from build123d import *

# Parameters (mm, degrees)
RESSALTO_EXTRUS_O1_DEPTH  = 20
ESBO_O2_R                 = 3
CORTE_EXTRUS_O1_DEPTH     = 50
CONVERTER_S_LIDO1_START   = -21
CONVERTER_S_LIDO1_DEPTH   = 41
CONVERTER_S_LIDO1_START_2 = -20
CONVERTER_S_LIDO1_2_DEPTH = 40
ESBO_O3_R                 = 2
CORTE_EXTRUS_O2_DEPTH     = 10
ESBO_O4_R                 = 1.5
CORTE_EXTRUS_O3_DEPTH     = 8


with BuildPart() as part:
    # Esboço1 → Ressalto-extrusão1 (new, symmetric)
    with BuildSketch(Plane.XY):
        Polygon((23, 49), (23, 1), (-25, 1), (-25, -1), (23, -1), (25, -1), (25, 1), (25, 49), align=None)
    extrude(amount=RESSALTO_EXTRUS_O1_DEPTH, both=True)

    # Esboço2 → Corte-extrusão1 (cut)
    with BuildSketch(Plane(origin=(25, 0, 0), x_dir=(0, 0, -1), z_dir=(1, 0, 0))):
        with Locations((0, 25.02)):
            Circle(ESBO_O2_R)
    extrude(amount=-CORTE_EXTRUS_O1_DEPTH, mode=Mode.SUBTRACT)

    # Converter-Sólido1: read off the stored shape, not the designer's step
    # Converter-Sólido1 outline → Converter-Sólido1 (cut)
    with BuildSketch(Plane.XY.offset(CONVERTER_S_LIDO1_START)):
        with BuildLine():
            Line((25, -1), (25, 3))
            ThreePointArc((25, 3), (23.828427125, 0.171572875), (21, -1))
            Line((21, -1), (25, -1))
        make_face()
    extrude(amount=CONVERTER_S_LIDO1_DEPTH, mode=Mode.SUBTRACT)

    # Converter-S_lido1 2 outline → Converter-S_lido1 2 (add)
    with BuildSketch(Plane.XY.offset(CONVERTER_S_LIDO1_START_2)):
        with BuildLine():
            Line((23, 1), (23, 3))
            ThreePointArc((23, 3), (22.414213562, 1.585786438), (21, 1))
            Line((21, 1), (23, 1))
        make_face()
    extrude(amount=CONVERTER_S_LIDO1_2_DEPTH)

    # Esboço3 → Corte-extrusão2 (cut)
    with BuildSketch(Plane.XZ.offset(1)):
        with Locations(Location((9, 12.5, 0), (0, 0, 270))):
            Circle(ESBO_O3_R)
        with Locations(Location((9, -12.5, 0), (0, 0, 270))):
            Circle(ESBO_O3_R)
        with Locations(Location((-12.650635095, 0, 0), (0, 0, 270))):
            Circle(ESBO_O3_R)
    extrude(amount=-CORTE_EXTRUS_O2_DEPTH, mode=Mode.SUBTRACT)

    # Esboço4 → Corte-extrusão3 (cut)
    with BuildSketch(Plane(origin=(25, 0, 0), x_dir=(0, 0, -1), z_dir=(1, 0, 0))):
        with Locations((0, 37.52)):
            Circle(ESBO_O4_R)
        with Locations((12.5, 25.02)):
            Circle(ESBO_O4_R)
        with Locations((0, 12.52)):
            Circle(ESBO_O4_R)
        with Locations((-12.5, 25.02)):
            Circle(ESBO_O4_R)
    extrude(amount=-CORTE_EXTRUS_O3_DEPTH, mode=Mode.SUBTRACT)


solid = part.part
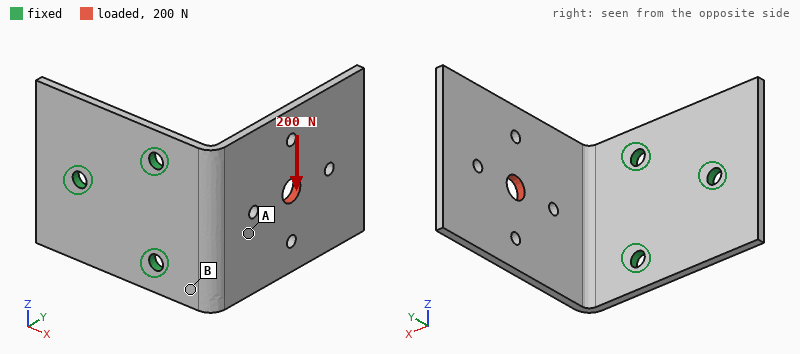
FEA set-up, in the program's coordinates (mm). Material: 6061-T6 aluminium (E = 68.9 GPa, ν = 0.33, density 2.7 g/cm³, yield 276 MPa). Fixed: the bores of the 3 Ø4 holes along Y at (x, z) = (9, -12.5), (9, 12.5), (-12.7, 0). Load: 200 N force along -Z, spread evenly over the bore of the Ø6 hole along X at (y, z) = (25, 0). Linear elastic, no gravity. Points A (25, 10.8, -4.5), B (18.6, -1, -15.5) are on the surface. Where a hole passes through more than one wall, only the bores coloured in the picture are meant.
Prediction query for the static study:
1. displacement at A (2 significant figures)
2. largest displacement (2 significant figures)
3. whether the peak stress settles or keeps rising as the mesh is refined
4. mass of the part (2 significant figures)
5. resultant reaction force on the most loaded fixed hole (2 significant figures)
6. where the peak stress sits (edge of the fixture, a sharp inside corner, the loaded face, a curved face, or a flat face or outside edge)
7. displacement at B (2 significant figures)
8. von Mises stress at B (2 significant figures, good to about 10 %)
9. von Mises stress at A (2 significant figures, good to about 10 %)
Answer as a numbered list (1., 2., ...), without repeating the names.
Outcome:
1. 0.086 mm
2. 0.42 mm
3. keeps rising
4. 20 g
5. 230 N
6. edge of the fixture
7. 0.064 mm
8. 43 MPa
9. 14 MPa
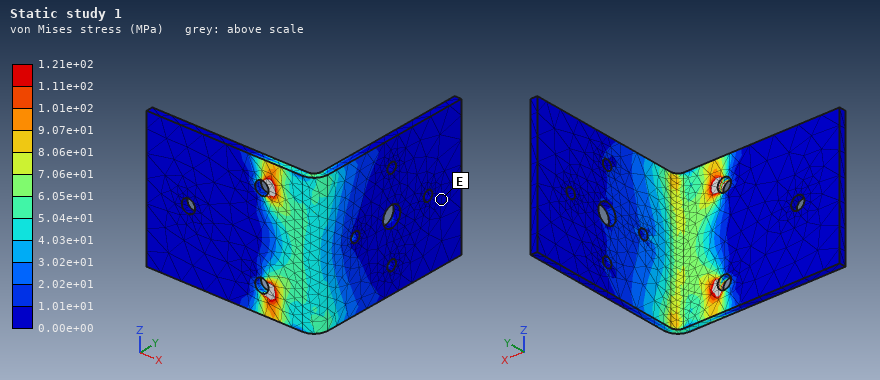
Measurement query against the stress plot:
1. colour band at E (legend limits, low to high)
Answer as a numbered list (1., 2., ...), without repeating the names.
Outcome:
1. 0.00e+00 to 1.01e+01 MPa
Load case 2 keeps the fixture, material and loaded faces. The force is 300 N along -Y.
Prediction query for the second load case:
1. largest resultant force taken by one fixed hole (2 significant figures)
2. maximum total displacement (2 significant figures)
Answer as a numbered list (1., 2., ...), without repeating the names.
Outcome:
1. 160 N
2. 0.82 mm
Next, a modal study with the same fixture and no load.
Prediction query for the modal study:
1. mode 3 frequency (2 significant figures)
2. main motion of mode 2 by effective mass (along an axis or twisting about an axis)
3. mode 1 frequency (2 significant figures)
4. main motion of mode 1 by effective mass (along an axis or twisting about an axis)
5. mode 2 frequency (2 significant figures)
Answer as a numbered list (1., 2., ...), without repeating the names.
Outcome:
1. 1900 Hz
2. along Z
3. 480 Hz
4. along X
5. 1200 Hz
